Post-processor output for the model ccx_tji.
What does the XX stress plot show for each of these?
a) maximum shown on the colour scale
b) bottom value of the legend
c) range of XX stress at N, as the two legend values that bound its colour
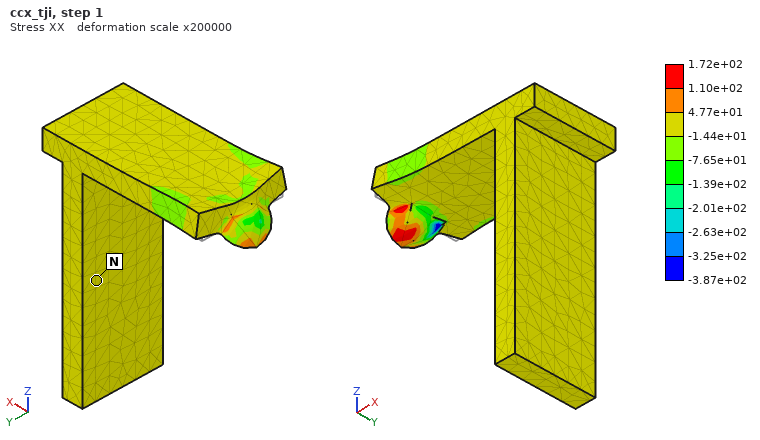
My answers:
1.72e+02
-3.87e+02
-1.44e+01 to 4.77e+01
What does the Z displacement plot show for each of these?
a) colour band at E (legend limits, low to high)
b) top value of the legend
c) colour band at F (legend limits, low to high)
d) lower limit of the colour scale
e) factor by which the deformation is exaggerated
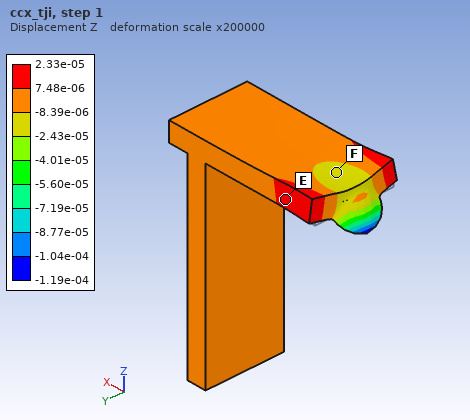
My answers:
7.48e-06 to 2.33e-05
2.33e-05
-2.43e-05 to -8.39e-06
-1.19e-04
200000
